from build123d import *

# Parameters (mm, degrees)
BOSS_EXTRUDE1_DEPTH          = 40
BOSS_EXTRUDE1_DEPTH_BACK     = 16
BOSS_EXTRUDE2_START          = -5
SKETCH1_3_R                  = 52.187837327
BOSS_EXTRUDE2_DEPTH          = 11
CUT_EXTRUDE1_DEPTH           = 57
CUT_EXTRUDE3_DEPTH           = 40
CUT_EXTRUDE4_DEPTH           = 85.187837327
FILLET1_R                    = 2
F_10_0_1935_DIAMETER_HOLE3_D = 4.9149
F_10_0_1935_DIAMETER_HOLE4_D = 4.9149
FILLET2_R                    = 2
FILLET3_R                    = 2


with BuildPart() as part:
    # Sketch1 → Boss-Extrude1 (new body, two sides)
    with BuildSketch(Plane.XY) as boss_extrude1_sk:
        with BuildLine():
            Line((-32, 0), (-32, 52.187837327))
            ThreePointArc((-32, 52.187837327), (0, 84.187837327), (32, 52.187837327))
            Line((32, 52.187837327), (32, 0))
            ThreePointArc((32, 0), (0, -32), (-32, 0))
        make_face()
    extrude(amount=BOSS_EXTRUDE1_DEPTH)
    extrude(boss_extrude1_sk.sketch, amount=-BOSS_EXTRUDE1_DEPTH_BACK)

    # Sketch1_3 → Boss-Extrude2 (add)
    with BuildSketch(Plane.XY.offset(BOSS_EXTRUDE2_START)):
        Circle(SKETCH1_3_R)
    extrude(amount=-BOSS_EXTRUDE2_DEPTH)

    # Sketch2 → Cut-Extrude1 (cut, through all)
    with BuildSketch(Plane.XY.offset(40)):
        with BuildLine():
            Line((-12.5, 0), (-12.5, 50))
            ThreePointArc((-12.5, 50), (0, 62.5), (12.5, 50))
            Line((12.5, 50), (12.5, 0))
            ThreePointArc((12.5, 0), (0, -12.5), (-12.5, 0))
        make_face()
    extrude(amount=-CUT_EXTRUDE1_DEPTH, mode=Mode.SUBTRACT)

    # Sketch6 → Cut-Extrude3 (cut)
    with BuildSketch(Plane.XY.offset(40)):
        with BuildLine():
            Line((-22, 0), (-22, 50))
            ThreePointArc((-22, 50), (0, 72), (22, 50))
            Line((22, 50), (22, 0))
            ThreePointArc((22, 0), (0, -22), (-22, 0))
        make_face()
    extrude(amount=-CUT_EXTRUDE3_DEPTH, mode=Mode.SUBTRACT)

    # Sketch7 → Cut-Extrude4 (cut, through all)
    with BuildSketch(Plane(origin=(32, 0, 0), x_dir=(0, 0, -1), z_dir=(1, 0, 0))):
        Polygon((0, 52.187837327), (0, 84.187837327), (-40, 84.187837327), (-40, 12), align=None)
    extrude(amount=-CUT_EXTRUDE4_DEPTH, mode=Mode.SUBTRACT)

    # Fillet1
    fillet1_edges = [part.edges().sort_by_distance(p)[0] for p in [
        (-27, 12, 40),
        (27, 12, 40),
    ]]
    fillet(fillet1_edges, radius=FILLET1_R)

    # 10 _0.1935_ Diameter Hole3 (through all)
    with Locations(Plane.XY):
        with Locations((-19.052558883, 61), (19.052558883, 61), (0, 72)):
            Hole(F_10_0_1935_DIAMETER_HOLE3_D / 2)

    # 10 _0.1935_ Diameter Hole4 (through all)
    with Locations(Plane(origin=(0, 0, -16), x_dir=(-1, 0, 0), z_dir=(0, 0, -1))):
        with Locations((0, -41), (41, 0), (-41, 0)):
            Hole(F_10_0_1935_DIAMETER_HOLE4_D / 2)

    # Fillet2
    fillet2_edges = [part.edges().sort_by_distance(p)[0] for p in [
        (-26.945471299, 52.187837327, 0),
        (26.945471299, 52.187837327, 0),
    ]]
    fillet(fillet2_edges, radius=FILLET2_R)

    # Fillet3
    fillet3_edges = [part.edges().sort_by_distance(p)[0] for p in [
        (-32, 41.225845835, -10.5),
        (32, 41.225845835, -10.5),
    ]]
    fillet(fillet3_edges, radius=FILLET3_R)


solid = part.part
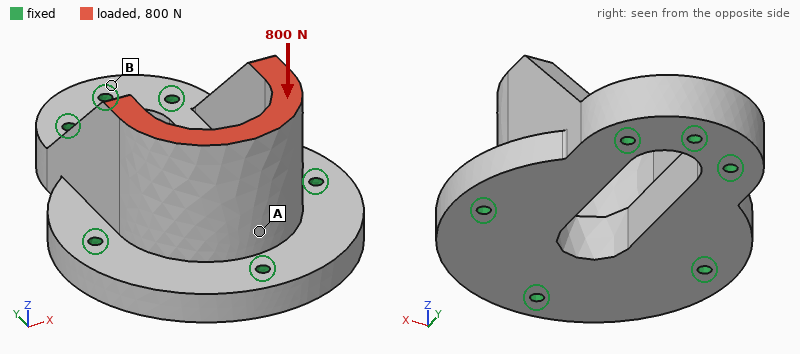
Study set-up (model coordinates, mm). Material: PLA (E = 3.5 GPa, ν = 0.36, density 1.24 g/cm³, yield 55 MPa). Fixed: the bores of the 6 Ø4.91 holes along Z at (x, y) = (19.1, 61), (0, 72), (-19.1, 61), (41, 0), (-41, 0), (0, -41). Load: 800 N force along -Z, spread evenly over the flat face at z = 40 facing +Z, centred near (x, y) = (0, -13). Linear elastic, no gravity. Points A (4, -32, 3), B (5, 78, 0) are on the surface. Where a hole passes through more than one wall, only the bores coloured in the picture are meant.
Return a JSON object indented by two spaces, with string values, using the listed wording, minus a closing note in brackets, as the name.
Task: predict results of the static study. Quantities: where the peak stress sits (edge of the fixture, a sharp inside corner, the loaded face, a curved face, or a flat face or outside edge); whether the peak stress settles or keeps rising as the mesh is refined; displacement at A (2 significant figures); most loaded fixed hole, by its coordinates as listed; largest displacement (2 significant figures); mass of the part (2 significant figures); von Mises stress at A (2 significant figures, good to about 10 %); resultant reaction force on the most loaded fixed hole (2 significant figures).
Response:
{
  "where the peak stress sits": "edge of the fixture",
  "whether the peak stress settles or keeps rising as the mesh is refined": "keeps rising",
  "displacement at A": "24 µm",
  "most loaded fixed hole, by its coordinates as listed": "(0, -41)",
  "largest displacement": "37 µm",
  "mass of the part": "220 g",
  "von Mises stress at A": "1.5 MPa",
  "resultant reaction force on the most loaded fixed hole": "340 N"
}
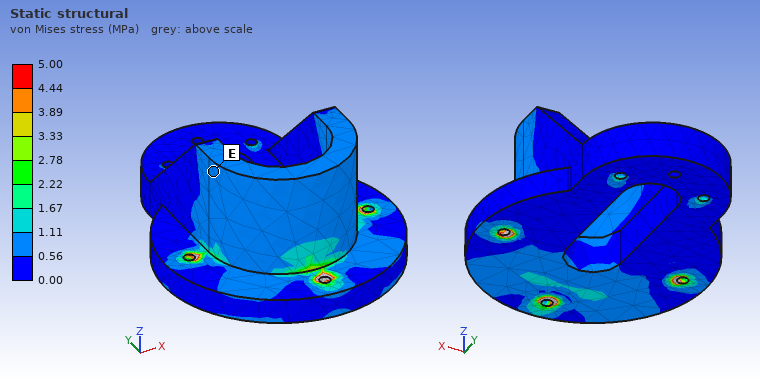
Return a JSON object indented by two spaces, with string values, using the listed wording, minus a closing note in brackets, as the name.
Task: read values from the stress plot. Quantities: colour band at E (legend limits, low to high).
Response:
{
  "colour band at E": "0.56 to 1.11 MPa"
}
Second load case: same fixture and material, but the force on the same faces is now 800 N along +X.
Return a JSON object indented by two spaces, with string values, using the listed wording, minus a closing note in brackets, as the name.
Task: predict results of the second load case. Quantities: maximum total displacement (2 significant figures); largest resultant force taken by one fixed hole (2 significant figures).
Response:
{
  "maximum total displacement": "0.24 mm",
  "largest resultant force taken by one fixed hole": "630 N"
}
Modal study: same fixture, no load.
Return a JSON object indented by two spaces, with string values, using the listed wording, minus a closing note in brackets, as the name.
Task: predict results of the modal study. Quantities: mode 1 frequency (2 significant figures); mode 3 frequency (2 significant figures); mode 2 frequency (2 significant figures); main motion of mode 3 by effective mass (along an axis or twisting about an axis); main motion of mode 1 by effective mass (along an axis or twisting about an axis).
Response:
{
  "mode 1 frequency": "1900 Hz",
  "mode 3 frequency": "2800 Hz",
  "mode 2 frequency": "2200 Hz",
  "main motion of mode 3 by effective mass": "along Z",
  "main motion of mode 1 by effective mass": "along X"
}
